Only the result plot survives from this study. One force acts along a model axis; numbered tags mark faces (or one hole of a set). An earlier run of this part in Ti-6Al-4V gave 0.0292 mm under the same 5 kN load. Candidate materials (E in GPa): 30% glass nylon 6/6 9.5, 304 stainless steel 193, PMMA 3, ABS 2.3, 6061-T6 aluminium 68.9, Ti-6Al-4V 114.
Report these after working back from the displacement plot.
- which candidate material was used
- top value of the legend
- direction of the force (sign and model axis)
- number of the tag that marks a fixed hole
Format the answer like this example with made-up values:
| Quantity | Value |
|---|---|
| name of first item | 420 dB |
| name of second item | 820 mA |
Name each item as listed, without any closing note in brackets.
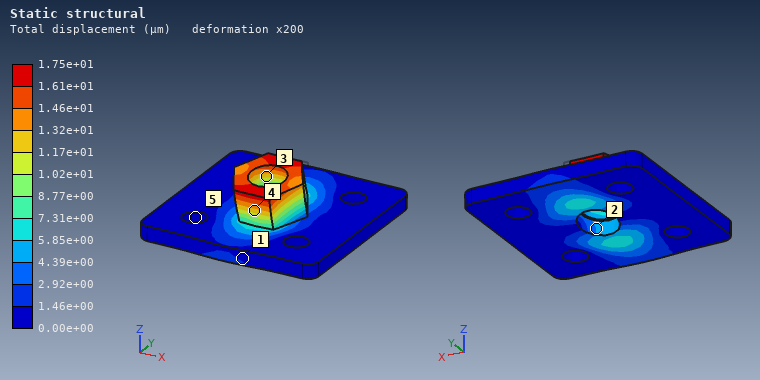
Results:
| Quantity | Value |
|---|---|
| which candidate material was used | 304 stainless steel |
| top value of the legend | 1.75e+01 µm |
| direction of the force | -Y |
| number of the tag that marks a fixed hole | 5 |
